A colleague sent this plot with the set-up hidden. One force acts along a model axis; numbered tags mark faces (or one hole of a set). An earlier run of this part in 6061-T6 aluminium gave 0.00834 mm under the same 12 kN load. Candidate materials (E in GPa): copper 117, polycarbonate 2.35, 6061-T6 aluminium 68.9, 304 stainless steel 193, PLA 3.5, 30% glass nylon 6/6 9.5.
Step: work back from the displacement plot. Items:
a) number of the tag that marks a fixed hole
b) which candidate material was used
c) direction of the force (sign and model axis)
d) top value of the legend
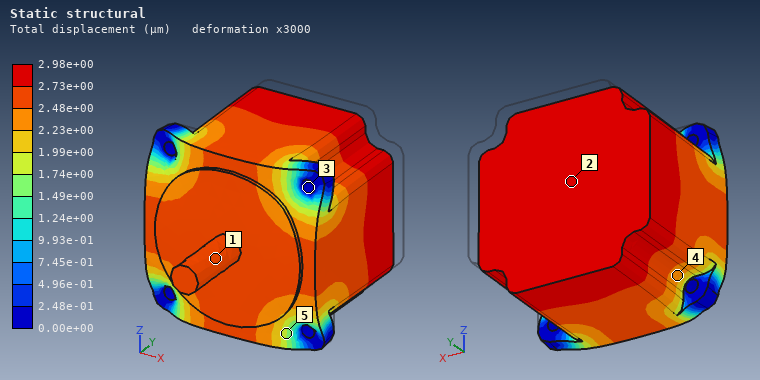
3
304 stainless steel
-Y
2.98e+00 µm
